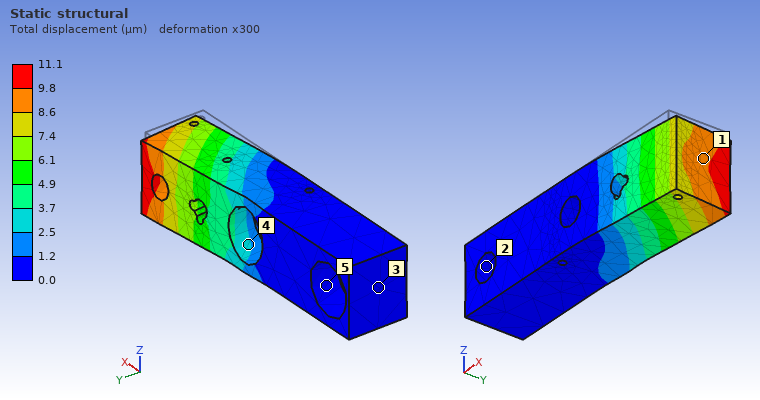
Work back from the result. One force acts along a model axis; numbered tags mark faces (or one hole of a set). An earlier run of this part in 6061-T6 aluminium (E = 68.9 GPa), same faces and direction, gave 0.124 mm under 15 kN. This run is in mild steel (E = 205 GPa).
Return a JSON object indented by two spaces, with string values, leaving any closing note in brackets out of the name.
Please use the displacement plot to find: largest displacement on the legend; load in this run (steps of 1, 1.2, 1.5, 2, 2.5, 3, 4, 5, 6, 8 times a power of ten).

{
  "largest displacement on the legend": "11.1 µm",
  "load in this run": "4 kN"
}
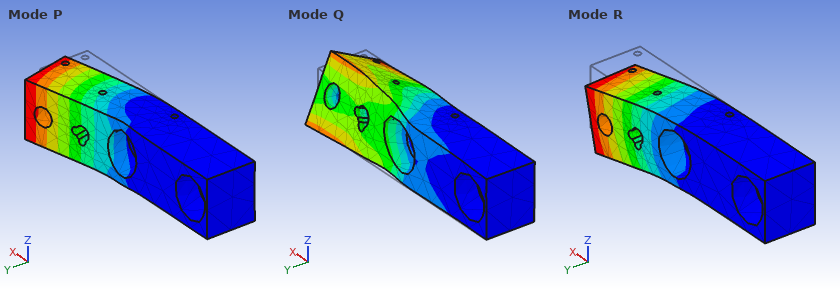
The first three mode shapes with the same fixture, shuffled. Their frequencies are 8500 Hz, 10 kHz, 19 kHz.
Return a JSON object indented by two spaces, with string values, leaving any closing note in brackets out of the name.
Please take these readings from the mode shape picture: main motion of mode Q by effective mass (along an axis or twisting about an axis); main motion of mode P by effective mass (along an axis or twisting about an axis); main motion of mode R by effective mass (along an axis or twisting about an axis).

{
  "main motion of mode Q by effective mass": "twisting about X",
  "main motion of mode P by effective mass": "along Y",
  "main motion of mode R by effective mass": "along Z"
}
